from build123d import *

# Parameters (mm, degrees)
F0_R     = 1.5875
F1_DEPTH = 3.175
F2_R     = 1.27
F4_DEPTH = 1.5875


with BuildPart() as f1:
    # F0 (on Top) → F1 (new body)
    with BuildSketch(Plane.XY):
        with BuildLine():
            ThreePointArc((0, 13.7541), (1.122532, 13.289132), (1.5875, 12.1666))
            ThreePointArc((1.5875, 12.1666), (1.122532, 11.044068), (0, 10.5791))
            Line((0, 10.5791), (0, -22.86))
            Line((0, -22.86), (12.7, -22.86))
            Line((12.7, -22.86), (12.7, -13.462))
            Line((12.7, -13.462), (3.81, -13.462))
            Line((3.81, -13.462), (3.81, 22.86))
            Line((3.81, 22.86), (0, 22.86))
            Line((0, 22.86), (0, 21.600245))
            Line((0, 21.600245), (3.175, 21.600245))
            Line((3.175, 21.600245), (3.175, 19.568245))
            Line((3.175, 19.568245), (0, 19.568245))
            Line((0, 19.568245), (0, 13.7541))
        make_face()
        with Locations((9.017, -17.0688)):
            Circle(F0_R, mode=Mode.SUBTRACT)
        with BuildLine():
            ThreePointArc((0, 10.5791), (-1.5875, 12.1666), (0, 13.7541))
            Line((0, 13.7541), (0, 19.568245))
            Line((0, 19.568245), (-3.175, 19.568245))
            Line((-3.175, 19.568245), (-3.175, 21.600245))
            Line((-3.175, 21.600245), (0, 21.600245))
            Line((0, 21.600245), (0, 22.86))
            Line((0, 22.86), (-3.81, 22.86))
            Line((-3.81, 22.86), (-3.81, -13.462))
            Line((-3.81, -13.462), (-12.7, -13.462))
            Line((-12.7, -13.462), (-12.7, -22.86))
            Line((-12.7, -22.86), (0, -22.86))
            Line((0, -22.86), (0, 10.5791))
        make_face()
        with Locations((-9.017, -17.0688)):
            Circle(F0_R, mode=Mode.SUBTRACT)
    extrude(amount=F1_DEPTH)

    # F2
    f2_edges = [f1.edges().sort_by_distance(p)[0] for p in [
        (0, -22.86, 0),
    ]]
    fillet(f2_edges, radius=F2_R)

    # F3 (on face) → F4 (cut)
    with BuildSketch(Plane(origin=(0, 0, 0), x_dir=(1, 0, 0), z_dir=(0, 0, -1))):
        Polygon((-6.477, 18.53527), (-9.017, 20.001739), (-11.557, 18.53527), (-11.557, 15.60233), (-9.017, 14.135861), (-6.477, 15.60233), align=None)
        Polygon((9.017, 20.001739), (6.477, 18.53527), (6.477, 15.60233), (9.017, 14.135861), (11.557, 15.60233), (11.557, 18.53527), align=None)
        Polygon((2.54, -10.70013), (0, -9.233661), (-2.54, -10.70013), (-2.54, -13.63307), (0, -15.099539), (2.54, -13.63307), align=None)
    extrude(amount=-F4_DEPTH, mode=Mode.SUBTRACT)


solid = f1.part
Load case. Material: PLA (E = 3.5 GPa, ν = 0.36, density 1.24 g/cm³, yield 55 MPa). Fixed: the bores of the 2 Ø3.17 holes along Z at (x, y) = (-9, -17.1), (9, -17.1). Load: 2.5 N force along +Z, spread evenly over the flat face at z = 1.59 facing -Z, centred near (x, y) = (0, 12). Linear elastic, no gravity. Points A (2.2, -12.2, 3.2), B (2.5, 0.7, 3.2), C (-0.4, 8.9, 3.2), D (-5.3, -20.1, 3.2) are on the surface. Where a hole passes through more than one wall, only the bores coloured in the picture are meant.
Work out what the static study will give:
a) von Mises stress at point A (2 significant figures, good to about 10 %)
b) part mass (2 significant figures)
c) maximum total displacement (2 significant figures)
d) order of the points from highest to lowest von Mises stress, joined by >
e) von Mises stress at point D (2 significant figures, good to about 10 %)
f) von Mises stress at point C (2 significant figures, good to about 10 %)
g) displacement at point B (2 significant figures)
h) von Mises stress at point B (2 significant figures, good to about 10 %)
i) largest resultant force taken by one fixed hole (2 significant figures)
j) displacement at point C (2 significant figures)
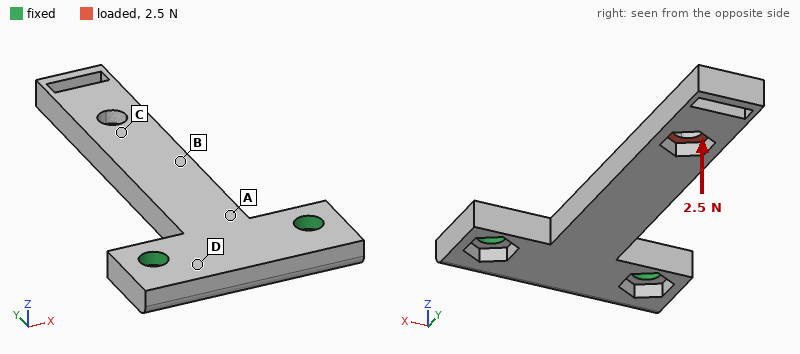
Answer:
4.7 MPa
1.8 g
0.55 mm
A > B > D > C
1.4 MPa
0.66 MPa
0.18 mm
2.2 MPa
4.2 N
0.31 mm
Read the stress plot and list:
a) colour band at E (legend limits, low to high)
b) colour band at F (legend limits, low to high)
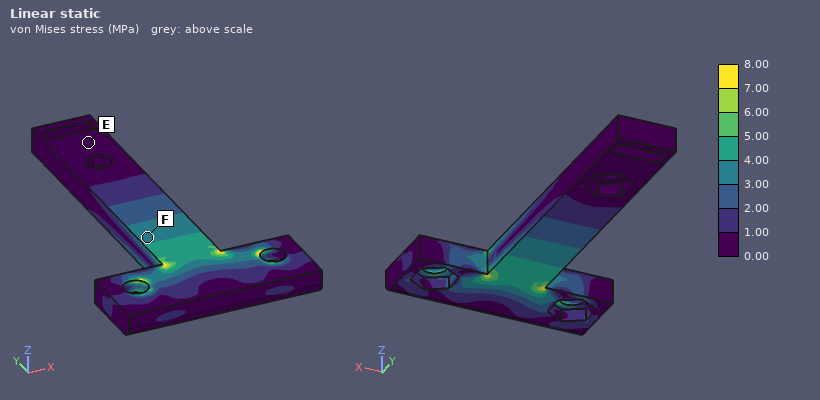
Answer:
0.00 to 1.00 MPa
3.00 to 4.00 MPa
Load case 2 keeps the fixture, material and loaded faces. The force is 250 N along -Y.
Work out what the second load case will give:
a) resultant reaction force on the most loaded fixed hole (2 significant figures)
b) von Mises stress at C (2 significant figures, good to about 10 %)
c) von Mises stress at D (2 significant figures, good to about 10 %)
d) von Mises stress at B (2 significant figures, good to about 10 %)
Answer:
130 N
6.1 MPa
8.7 MPa
10 MPa
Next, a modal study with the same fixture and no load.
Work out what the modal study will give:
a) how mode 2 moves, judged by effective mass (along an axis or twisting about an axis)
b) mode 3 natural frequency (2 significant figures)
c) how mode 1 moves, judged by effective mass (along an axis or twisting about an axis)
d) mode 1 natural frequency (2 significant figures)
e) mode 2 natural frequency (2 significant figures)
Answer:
along X
2900 Hz
along Z
550 Hz
1500 Hz
